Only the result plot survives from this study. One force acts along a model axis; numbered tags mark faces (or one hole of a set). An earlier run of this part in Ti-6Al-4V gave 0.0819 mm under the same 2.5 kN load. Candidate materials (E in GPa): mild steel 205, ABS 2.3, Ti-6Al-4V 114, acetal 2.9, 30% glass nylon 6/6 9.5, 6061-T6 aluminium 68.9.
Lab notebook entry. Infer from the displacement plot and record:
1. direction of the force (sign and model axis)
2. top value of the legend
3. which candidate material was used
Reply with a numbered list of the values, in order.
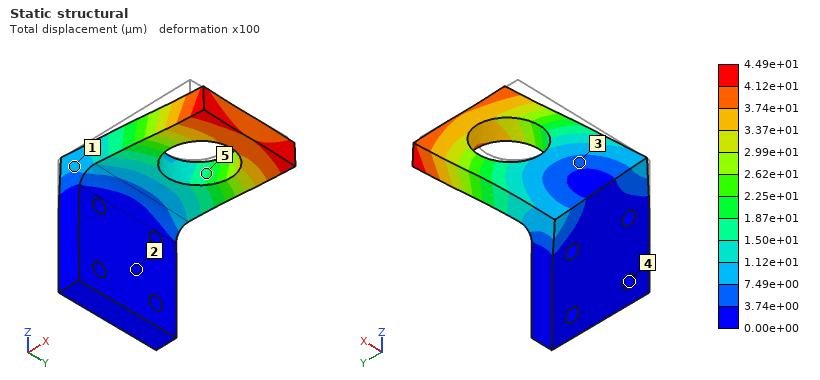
1. +Y
2. 4.49e+01 µm
3. mild steel
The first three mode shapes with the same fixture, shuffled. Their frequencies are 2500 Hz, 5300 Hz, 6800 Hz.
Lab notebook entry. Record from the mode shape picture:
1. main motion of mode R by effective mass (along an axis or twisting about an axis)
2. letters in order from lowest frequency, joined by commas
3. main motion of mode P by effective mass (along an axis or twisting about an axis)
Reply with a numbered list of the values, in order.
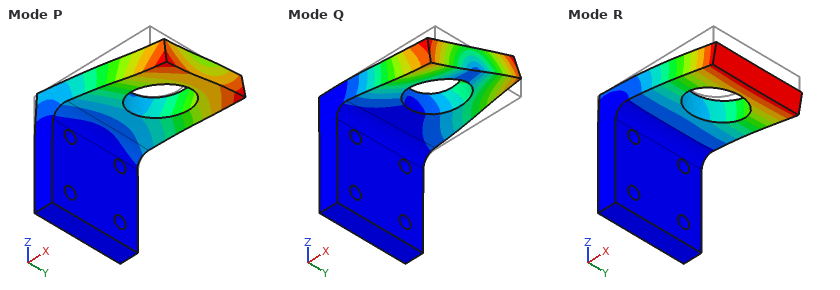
1. along Z
2. R, P, Q
3. along Y
